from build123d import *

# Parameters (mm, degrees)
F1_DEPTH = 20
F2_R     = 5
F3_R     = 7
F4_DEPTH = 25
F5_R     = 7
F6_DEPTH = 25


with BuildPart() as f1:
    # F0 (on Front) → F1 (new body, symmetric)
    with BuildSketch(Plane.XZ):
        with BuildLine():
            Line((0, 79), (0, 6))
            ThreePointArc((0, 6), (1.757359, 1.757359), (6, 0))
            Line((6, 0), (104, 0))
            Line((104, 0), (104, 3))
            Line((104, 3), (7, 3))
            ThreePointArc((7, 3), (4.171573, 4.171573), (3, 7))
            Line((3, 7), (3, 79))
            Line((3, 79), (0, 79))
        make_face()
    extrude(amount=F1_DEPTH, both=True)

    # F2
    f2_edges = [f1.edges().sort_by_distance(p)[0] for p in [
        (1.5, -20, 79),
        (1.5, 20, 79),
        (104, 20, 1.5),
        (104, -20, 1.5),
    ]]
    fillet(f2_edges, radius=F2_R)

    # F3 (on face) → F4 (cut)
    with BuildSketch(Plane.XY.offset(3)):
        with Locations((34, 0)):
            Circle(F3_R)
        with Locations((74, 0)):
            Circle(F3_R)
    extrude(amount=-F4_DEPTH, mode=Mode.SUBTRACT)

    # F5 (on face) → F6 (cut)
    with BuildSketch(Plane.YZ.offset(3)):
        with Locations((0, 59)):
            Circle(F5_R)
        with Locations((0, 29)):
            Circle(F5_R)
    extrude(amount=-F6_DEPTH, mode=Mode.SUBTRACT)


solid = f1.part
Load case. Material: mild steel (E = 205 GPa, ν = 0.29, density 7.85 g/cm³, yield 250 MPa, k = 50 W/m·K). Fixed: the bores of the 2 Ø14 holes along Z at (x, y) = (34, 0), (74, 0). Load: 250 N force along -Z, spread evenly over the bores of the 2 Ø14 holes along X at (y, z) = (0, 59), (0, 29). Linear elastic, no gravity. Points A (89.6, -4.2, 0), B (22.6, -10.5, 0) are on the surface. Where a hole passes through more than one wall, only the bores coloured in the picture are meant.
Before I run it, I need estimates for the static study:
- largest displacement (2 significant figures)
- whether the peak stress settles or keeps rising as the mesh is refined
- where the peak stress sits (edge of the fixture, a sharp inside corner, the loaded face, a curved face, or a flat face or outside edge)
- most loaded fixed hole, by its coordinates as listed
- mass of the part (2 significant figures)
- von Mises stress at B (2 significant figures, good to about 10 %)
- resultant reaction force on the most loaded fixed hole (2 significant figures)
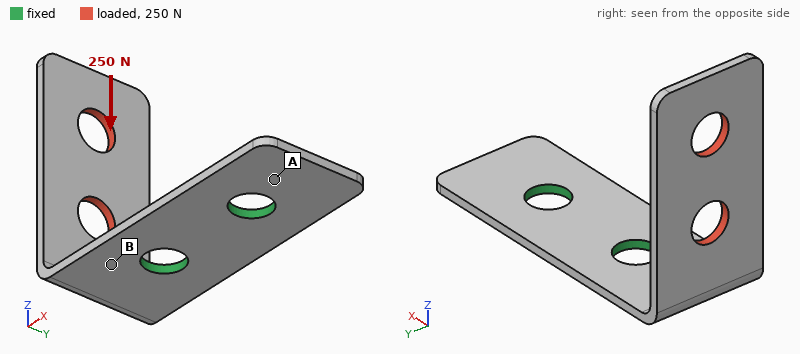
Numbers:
0.40 mm
keeps rising
edge of the fixture
(34, 0)
150 g
76 MPa
260 N
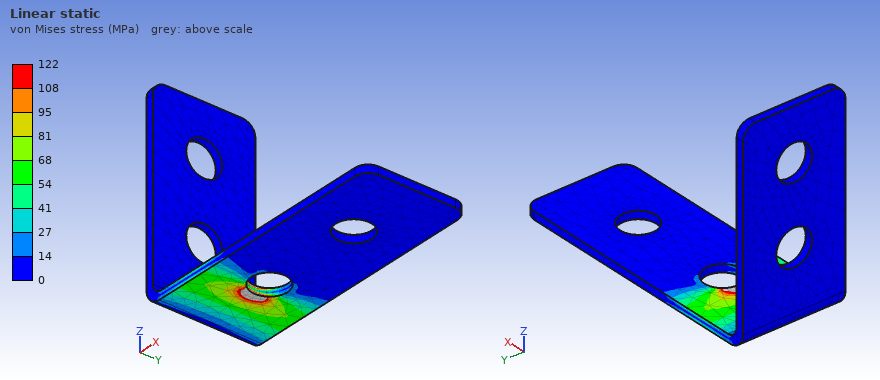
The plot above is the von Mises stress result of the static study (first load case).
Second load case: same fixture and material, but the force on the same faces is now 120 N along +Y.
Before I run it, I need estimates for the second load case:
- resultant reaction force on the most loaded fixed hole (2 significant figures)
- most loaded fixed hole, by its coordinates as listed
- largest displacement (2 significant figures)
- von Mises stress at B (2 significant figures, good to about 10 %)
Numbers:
160 N
(34, 0)
0.29 mm
43 MPa
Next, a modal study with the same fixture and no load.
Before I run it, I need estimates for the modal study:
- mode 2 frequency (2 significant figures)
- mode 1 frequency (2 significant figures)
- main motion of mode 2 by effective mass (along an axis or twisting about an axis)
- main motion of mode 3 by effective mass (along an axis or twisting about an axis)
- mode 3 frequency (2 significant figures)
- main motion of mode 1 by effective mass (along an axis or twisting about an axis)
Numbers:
500 Hz
280 Hz
along Y
along Z
1200 Hz
along X
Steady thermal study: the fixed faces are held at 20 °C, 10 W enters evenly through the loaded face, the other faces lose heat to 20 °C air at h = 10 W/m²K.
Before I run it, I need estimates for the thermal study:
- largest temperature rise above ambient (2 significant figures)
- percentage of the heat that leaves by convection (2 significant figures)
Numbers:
82 K
41 %
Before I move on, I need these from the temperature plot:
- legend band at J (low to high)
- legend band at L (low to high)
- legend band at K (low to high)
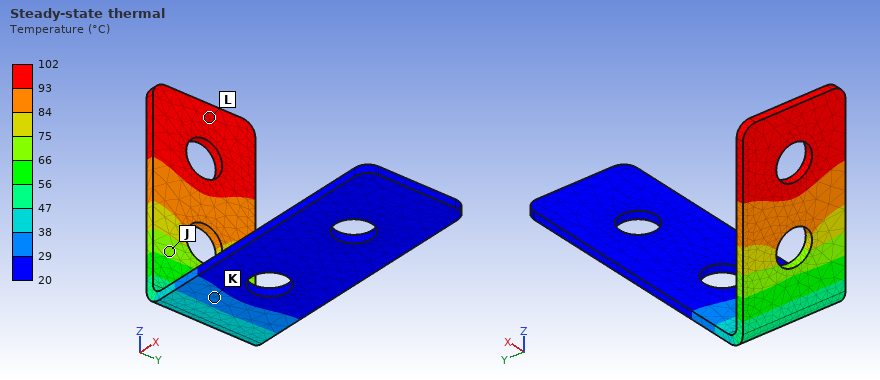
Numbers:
66 to 75 °C
93 to 102 °C
29 to 38 °C
